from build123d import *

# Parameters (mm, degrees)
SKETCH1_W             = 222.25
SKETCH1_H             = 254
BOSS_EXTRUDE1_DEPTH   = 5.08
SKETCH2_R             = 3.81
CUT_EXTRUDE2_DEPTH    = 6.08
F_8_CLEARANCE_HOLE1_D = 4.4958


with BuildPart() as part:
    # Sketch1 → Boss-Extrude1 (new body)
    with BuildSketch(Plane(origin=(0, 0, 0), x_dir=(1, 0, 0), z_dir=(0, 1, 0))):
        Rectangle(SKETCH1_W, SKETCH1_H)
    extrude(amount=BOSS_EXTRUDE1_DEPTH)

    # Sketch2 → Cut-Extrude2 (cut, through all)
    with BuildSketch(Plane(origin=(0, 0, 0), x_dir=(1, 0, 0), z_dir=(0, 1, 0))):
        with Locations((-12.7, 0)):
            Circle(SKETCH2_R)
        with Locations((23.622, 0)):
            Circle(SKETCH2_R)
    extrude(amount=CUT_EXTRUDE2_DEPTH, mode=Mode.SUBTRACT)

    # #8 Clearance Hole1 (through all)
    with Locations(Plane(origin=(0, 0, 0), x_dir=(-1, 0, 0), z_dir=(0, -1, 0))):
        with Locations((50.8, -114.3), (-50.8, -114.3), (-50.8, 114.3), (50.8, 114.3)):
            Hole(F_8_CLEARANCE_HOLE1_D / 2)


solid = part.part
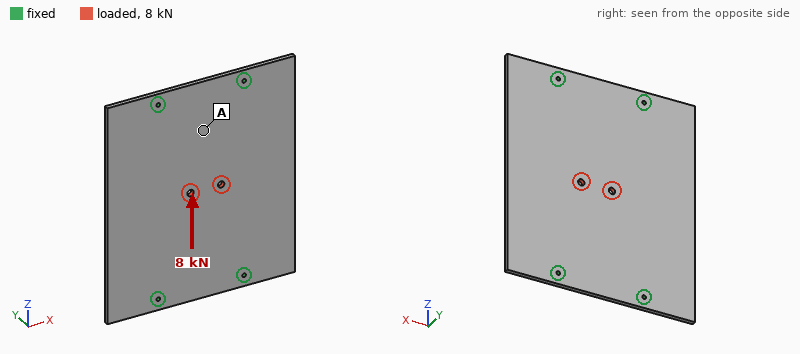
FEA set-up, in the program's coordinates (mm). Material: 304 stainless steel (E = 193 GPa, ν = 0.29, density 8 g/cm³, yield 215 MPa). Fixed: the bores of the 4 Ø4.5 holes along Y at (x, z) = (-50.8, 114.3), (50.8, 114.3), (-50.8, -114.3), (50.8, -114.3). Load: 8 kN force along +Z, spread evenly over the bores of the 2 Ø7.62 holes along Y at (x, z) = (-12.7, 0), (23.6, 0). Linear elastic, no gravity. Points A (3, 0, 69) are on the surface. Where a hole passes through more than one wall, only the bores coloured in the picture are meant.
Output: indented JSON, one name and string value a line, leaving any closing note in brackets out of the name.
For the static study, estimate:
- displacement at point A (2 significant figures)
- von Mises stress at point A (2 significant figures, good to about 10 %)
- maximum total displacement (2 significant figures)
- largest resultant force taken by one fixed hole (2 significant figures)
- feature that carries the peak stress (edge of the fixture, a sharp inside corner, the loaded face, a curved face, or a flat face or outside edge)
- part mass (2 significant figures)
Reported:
{
  "displacement at point A": "3.4 µm",
  "von Mises stress at point A": "5.2 MPa",
  "maximum total displacement": "7.0 µm",
  "largest resultant force taken by one fixed hole": "2.1 kN",
  "feature that carries the peak stress": "the loaded face",
  "part mass": "2.3 kg"
}
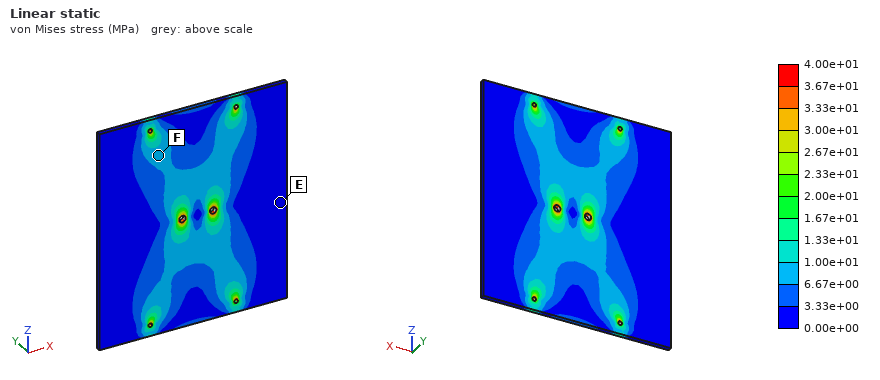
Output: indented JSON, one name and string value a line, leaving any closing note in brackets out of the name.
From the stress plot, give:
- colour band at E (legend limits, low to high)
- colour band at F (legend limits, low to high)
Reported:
{
  "colour band at E": "0.00e+00 to 3.33e+00 MPa",
  "colour band at F": "6.67e+00 to 1.00e+01 MPa"
}
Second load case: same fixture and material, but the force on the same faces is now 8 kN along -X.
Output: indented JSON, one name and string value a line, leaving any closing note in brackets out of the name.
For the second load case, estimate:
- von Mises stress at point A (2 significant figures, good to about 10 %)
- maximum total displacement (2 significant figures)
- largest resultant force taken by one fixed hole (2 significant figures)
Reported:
{
  "von Mises stress at point A": "9.0 MPa",
  "maximum total displacement": "12 µm",
  "largest resultant force taken by one fixed hole": "2.1 kN"
}
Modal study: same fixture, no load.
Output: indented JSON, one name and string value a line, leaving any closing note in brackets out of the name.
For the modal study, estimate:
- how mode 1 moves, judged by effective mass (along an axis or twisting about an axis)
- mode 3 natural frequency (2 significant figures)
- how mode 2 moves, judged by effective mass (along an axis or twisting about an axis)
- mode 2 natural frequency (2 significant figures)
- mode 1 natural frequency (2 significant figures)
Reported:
{
  "how mode 1 moves, judged by effective mass": "along Y",
  "mode 3 natural frequency": "720 Hz",
  "how mode 2 moves, judged by effective mass": "twisting about Z",
  "mode 2 natural frequency": "420 Hz",
  "mode 1 natural frequency": "380 Hz"
}
